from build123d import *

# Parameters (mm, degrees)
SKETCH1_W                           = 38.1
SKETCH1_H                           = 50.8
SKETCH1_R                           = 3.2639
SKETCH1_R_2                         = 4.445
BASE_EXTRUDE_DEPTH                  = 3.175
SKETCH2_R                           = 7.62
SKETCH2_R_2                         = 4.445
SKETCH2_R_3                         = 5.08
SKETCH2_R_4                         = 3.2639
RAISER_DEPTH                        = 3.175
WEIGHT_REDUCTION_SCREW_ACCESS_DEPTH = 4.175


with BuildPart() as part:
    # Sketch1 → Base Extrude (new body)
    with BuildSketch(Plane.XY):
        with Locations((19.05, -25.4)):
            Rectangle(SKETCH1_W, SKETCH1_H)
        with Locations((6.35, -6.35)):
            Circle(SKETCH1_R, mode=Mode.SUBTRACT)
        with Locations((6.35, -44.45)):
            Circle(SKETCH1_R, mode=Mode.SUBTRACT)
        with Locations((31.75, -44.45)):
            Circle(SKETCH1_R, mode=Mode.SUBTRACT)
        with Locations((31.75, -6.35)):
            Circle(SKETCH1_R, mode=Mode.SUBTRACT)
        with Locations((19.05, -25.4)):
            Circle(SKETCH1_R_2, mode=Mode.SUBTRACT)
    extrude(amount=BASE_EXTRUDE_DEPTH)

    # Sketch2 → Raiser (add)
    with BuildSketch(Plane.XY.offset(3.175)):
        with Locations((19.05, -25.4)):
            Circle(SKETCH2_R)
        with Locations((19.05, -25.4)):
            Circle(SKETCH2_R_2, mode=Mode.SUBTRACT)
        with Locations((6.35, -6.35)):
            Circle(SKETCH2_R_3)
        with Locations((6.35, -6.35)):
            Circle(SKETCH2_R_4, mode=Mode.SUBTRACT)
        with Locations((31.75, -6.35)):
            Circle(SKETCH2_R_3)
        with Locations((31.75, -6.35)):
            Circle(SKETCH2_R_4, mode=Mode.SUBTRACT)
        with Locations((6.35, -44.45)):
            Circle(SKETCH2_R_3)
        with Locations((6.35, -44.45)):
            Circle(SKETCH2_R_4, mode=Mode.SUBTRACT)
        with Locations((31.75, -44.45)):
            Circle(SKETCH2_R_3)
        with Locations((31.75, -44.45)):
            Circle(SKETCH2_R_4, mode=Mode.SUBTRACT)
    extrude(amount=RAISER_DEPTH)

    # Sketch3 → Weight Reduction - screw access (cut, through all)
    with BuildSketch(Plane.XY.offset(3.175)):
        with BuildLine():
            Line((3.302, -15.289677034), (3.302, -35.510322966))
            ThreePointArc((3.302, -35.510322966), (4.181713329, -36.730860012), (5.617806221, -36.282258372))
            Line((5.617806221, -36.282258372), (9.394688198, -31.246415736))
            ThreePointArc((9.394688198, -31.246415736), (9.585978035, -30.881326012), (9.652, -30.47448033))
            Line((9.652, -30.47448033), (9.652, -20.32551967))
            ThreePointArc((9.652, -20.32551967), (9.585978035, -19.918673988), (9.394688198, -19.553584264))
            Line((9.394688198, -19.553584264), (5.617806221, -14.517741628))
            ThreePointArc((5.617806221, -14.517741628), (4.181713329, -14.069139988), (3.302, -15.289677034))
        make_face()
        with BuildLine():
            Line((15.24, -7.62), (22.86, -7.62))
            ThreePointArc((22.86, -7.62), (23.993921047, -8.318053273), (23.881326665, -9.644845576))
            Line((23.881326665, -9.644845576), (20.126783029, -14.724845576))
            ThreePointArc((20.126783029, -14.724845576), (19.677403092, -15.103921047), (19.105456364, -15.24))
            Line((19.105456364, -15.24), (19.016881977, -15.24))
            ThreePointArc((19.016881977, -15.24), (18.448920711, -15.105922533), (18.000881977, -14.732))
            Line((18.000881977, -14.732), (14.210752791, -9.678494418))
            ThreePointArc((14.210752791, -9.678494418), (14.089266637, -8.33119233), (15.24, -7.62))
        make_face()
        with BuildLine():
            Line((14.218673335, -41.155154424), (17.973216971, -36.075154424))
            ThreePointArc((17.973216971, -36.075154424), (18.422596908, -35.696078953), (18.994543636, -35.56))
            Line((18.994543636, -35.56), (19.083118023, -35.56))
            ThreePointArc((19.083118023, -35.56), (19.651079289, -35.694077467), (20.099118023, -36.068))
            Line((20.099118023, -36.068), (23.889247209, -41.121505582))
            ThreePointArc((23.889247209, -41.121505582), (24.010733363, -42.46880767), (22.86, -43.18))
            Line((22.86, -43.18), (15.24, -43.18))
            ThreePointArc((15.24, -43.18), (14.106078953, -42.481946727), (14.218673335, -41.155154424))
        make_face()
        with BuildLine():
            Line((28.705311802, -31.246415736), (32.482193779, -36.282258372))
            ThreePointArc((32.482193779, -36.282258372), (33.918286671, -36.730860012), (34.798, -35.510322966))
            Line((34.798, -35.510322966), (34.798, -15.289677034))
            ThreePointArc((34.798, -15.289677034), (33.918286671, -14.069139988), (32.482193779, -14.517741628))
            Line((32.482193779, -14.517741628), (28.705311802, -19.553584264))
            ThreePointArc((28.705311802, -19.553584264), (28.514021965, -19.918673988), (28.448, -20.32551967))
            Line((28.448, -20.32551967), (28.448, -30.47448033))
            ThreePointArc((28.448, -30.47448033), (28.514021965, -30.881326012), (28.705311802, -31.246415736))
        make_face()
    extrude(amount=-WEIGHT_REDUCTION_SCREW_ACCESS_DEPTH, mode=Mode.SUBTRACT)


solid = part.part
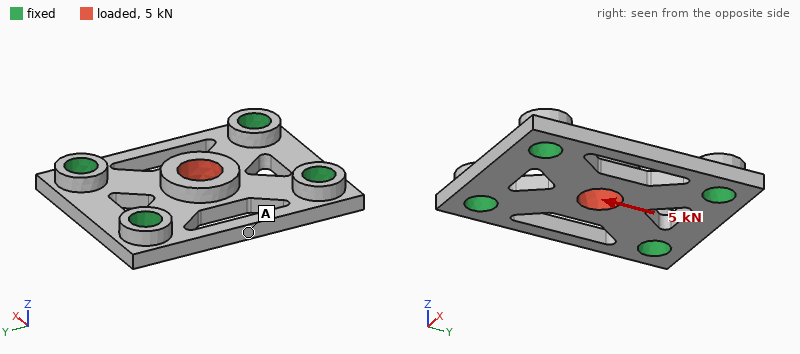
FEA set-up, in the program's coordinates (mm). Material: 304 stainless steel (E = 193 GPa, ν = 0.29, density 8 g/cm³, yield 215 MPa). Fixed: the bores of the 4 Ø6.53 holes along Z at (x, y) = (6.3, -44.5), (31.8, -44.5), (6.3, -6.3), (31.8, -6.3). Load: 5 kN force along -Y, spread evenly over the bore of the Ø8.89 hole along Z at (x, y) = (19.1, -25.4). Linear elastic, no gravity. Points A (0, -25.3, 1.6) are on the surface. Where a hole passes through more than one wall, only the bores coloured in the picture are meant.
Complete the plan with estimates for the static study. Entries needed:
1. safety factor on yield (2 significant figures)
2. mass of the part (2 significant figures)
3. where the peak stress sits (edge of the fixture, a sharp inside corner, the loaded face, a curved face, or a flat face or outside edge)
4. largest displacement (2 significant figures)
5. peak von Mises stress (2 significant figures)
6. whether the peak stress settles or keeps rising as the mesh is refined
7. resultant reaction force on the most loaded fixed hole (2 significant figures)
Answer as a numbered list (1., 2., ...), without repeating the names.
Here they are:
1. 1.5
2. 44 g
3. a curved face
4. 9.1 µm
5. 150 MPa
6. settles
7. 1.4 kN
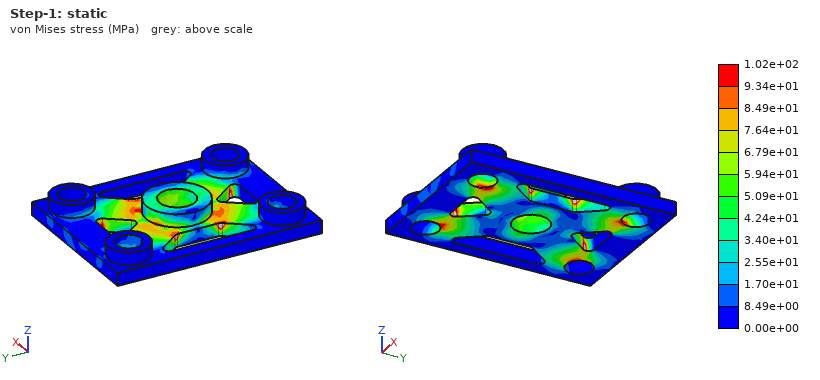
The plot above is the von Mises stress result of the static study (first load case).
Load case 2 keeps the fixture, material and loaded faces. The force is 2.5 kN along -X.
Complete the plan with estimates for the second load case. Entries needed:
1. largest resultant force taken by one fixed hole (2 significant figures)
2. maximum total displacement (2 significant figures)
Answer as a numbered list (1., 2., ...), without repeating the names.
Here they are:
1. 800 N
2. 8.4 µm
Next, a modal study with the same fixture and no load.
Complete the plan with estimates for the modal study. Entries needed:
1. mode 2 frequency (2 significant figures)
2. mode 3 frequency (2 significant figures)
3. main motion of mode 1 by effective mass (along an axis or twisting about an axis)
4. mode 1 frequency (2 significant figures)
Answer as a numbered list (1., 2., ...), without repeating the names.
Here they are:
1. 17 kHz
2. 17 kHz
3. along Z
4. 14 kHz
